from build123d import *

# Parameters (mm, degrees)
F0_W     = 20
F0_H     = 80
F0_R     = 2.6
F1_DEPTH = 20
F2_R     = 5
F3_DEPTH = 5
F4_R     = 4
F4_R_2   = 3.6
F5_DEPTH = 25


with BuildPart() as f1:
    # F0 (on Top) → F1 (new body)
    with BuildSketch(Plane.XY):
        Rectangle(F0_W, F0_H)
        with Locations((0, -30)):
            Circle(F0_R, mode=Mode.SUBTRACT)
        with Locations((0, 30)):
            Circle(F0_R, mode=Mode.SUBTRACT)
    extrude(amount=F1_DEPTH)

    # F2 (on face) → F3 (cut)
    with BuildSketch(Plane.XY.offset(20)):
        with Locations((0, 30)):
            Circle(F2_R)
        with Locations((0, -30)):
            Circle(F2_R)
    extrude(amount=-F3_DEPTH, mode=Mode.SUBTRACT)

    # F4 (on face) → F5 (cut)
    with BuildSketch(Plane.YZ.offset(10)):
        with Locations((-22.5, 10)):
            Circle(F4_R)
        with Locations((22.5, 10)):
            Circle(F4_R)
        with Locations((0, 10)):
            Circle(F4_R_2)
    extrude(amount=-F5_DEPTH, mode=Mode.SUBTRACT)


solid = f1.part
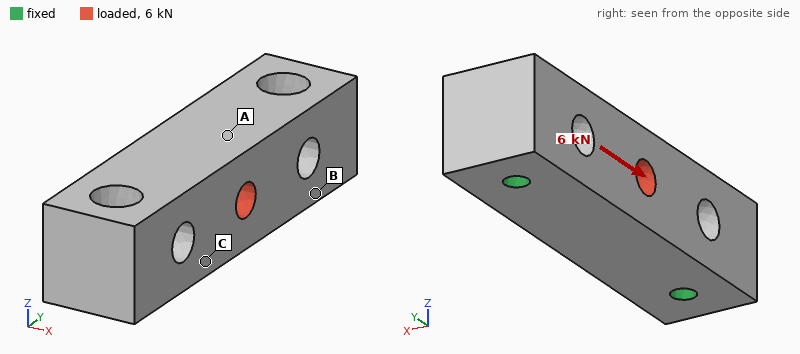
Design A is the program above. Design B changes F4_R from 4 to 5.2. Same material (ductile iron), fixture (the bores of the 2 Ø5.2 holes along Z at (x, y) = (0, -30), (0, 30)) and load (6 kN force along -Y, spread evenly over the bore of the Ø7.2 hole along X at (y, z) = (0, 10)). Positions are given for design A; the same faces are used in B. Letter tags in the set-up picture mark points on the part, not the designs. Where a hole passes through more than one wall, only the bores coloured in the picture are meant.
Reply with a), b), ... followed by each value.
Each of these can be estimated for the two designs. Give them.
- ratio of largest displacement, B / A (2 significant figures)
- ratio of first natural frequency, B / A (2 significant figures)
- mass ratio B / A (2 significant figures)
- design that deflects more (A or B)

a) 1.2
b) 0.91
c) 0.95
d) B
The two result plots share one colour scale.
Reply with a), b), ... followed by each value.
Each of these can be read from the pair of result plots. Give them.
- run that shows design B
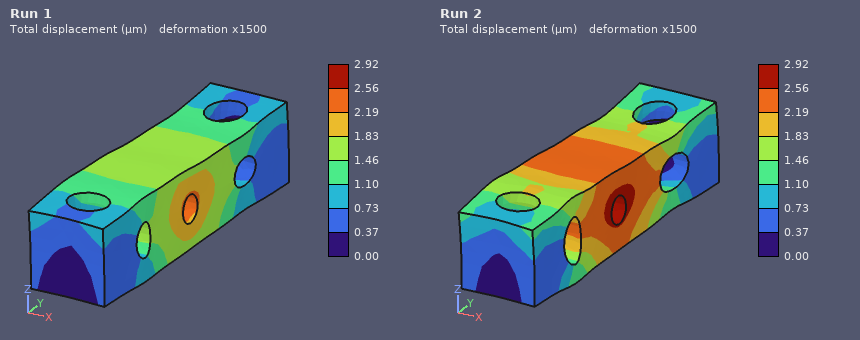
a) Run 2
